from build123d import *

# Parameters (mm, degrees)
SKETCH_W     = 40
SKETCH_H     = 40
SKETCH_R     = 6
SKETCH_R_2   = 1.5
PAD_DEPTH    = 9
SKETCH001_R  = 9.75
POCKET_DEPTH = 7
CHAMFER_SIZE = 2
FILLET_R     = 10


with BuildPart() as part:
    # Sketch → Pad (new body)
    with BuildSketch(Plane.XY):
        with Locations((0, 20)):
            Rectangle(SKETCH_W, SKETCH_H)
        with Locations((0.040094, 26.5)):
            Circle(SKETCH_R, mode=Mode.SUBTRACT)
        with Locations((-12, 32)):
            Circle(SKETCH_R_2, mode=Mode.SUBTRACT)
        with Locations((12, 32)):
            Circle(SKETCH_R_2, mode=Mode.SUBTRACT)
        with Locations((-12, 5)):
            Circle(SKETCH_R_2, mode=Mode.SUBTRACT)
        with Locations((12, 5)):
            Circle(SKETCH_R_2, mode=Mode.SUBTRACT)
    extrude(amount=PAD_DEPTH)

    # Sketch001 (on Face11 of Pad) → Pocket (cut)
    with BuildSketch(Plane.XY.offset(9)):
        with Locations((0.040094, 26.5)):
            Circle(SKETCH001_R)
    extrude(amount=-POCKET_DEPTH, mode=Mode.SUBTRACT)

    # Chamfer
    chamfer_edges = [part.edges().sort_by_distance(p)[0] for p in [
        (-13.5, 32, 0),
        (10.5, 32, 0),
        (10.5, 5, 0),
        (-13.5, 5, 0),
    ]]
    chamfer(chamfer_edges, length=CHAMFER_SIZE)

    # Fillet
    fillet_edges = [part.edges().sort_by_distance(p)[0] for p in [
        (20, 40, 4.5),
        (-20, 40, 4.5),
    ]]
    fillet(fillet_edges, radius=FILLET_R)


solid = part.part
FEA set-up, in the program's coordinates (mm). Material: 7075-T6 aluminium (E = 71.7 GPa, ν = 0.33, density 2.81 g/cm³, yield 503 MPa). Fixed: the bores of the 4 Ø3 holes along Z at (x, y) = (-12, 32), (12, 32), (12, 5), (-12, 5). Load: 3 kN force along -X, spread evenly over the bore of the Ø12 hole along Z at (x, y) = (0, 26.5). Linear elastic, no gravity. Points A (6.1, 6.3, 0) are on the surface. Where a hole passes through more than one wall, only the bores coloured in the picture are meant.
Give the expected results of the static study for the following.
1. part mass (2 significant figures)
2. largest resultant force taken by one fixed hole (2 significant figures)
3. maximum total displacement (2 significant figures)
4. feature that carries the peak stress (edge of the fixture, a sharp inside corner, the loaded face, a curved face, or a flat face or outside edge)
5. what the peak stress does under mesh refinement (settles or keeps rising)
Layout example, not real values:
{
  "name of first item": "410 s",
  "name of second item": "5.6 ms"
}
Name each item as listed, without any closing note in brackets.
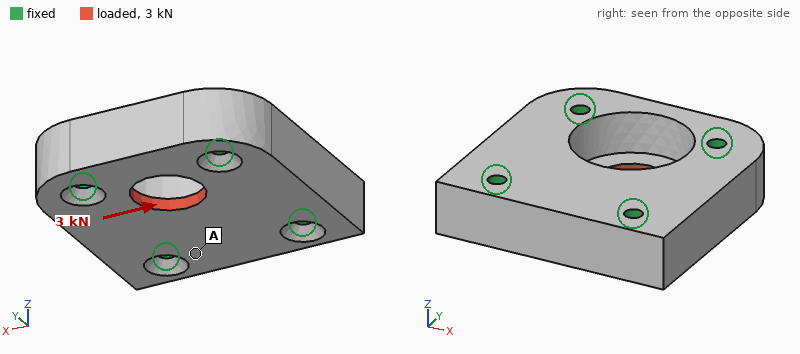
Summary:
{
  "part mass": "32 g",
  "largest resultant force taken by one fixed hole": "1.0 kN",
  "maximum total displacement": "8.2 µm",
  "feature that carries the peak stress": "edge of the fixture",
  "what the peak stress does under mesh refinement": "keeps rising"
}
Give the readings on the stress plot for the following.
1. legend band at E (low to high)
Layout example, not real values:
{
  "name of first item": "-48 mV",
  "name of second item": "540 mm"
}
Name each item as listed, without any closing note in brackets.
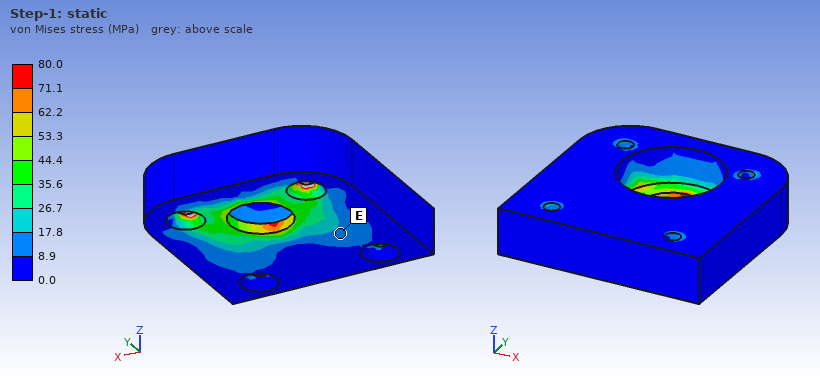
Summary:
{
  "legend band at E": "8.9 to 17.8 MPa"
}
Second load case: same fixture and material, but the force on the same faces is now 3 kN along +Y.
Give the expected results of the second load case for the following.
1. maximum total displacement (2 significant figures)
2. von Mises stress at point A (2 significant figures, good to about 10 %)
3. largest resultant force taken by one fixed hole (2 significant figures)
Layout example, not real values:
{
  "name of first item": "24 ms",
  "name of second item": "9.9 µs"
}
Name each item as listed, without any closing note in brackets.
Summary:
{
  "maximum total displacement": "12 µm",
  "von Mises stress at point A": "8.0 MPa",
  "largest resultant force taken by one fixed hole": "970 N"
}
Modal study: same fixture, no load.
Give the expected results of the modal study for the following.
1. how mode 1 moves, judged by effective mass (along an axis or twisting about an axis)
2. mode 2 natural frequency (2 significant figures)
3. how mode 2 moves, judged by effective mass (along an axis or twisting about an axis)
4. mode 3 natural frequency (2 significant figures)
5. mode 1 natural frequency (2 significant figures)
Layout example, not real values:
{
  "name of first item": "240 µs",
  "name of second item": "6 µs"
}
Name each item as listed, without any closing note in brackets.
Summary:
{
  "how mode 1 moves, judged by effective mass": "along Z",
  "mode 2 natural frequency": "34 kHz",
  "how mode 2 moves, judged by effective mass": "twisting about Y",
  "mode 3 natural frequency": "36 kHz",
  "mode 1 natural frequency": "29 kHz"
}
